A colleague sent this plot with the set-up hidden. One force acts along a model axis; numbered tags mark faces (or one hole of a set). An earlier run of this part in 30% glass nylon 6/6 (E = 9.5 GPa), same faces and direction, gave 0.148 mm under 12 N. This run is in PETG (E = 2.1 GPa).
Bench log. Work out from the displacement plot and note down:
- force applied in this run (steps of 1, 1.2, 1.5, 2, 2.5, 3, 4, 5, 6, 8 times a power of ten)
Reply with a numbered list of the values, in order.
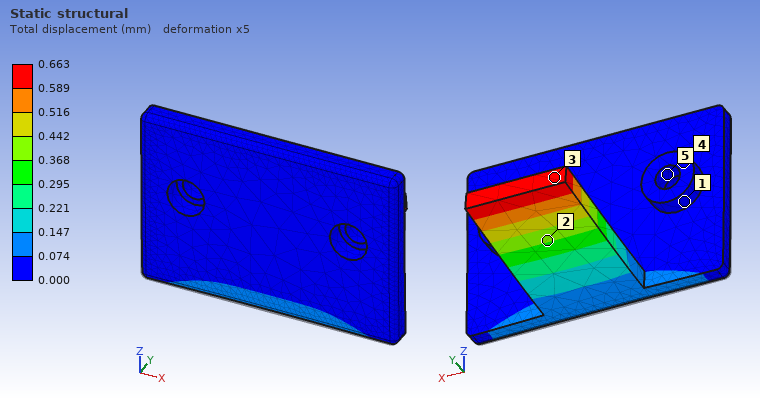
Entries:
1. 12 N
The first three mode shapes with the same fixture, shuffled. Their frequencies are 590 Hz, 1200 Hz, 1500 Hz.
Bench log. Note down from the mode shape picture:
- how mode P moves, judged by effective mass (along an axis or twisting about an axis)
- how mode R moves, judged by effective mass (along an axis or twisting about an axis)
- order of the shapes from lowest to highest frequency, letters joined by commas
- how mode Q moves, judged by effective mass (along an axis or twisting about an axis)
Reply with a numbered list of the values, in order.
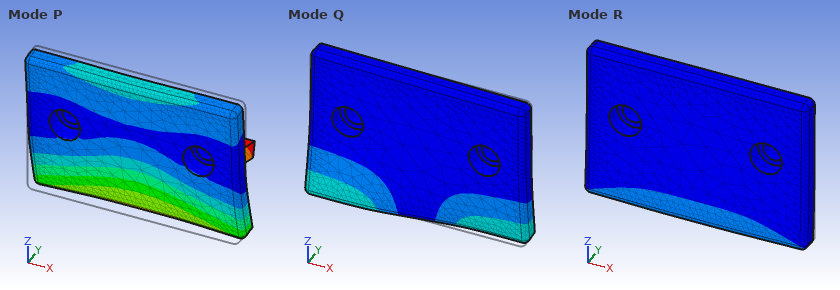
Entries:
1. along Y
2. along Z
3. R, Q, P
4. along X
